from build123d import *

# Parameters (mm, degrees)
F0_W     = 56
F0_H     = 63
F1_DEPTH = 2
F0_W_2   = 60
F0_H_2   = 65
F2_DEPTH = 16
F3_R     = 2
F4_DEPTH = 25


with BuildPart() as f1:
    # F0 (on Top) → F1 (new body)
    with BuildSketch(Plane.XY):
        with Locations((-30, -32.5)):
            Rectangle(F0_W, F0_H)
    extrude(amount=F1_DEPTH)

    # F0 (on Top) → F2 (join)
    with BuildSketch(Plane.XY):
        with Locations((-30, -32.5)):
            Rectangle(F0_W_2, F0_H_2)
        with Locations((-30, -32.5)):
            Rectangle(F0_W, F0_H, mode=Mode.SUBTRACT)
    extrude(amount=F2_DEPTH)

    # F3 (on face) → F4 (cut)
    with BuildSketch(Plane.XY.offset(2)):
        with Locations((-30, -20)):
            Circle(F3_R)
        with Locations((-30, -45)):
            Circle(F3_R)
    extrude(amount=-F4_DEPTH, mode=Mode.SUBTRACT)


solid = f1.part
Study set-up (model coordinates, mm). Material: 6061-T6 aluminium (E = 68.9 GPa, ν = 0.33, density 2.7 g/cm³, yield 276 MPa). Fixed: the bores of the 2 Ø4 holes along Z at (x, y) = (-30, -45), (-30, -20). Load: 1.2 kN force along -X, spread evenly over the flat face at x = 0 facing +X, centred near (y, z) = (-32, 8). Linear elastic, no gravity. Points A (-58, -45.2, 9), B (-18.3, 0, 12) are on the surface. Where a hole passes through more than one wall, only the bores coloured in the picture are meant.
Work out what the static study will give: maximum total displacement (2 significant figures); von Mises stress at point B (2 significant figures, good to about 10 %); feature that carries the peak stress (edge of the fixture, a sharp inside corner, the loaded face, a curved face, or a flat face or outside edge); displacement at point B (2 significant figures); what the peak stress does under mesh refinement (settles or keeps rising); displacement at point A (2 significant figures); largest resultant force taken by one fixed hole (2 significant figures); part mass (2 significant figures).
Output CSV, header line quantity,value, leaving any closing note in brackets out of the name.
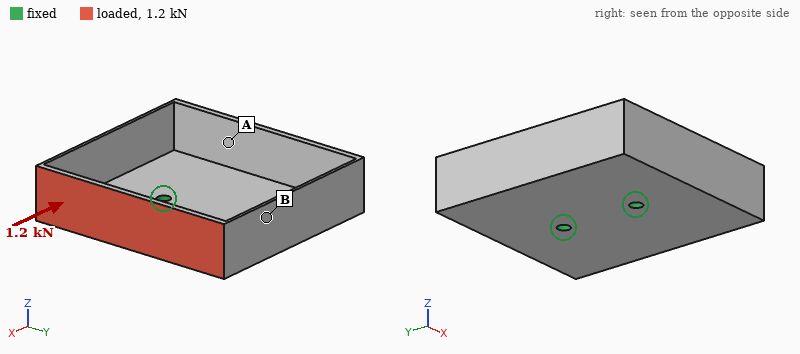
quantity,value
maximum total displacement,0.88 mm
von Mises stress at point B,49 MPa
feature that carries the peak stress,edge of the fixture
displacement at point B,0.32 mm
what the peak stress does under mesh refinement,keeps rising
displacement at point A,0.43 mm
largest resultant force taken by one fixed hole,610 N
part mass,35 g
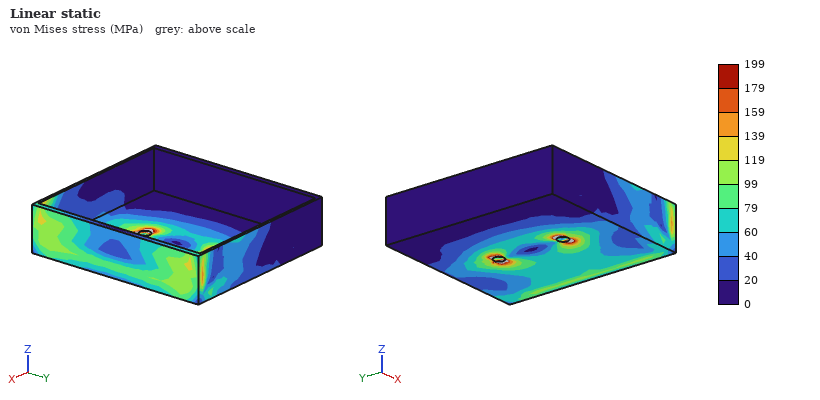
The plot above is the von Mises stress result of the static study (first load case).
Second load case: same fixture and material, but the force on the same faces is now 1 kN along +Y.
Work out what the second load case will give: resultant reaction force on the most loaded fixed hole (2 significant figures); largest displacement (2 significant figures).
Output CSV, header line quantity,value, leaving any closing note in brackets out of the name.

quantity,value
resultant reaction force on the most loaded fixed hole,1.2 kN
largest displacement,0.57 mm
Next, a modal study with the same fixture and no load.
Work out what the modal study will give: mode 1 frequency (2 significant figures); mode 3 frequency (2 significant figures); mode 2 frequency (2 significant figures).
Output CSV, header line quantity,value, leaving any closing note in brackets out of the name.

quantity,value
mode 1 frequency,950 Hz
mode 3 frequency,1700 Hz
mode 2 frequency,1300 Hz
